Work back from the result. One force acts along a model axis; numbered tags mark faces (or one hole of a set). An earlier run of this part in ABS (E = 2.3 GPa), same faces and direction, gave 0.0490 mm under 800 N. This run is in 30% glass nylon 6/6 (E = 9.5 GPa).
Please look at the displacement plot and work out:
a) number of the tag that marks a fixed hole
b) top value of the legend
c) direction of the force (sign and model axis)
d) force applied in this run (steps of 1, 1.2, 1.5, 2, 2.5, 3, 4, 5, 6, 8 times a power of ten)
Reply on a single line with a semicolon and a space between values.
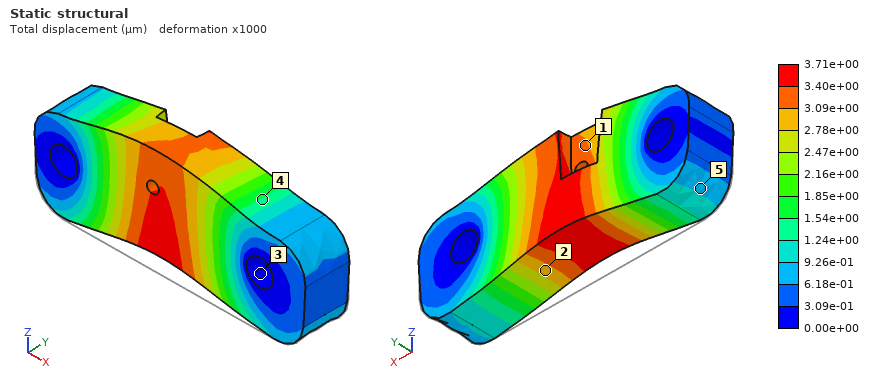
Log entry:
3; 3.71e+00 µm; +Z; 250 N
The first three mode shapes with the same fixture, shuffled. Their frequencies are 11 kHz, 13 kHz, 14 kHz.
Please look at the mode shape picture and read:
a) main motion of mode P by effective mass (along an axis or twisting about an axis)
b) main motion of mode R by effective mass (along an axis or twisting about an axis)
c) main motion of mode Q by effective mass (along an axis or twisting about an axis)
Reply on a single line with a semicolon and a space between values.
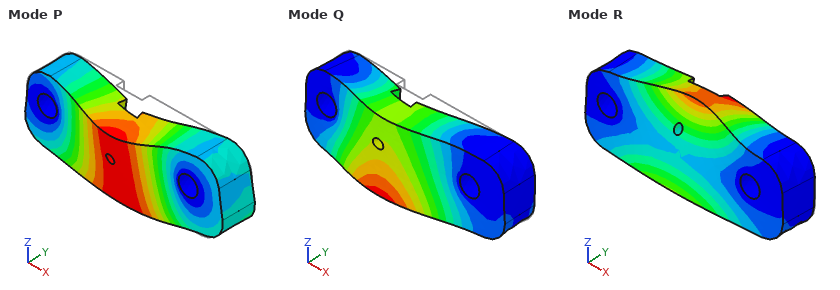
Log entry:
along Z; twisting about X; along Y
